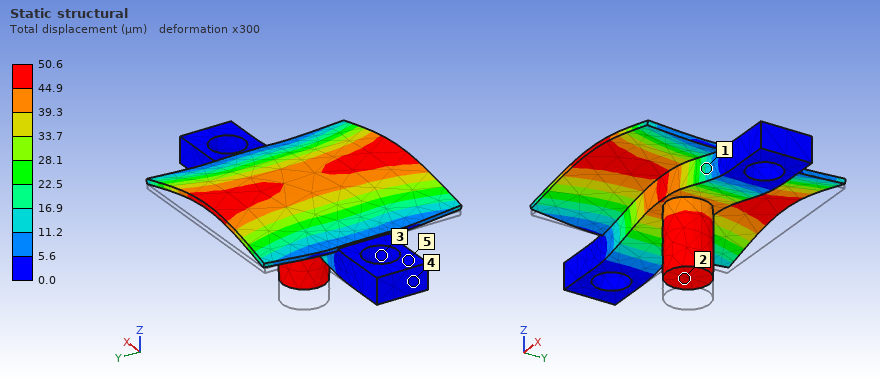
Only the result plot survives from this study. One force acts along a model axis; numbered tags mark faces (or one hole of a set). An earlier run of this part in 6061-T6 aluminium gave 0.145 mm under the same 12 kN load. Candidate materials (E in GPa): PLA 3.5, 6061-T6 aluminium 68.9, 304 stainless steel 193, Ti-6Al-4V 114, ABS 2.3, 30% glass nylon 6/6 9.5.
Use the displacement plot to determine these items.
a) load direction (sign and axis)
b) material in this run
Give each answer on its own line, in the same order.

+Z
304 stainless steel
